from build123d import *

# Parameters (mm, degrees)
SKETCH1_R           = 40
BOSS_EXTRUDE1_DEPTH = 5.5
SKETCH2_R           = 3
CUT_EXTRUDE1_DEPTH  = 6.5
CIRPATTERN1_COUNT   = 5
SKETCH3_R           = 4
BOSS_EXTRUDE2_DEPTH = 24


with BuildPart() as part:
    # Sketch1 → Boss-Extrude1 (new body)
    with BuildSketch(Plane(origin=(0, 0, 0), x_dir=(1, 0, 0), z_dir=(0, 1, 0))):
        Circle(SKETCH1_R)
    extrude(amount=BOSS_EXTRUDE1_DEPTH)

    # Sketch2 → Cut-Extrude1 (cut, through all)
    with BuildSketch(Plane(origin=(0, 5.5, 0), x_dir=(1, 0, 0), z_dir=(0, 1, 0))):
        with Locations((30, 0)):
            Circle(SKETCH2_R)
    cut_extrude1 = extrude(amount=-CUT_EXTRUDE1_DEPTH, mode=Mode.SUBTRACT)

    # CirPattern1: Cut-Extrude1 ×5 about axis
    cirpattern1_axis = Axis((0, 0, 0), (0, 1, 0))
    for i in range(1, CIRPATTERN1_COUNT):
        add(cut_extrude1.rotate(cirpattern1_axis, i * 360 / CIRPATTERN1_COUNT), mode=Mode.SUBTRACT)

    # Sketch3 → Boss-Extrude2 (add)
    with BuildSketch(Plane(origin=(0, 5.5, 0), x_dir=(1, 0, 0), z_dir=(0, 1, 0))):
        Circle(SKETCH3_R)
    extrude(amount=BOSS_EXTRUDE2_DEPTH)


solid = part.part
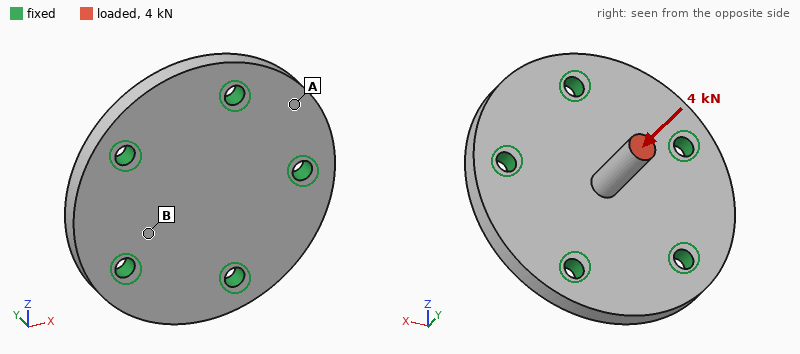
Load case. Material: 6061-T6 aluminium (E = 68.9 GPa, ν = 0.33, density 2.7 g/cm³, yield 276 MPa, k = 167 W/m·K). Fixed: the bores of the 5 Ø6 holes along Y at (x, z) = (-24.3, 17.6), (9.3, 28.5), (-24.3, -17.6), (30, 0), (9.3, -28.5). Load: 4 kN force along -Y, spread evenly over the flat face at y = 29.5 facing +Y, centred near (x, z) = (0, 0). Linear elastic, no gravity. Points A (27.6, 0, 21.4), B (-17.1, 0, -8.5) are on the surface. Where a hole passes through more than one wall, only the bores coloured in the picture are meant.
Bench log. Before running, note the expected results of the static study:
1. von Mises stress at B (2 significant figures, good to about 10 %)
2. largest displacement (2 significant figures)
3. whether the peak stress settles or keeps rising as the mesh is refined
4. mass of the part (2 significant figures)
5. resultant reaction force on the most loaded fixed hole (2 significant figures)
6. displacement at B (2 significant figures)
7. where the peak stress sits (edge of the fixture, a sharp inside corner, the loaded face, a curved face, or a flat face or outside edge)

32 MPa
0.10 mm
keeps rising
76 g
800 N
0.022 mm
edge of the fixture
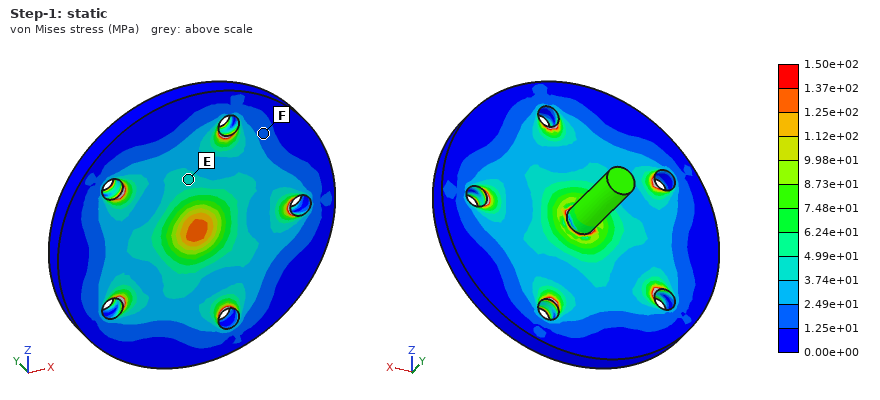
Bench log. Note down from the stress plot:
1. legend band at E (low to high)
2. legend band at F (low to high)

3.74e+01 to 4.99e+01 MPa
1.25e+01 to 2.49e+01 MPa
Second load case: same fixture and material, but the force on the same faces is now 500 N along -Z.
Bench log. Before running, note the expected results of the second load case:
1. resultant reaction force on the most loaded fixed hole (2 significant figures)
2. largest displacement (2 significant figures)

270 N
0.26 mm
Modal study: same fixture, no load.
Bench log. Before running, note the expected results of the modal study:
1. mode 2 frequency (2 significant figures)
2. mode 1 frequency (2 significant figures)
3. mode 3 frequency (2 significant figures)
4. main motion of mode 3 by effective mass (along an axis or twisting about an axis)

7300 Hz
7300 Hz
11 kHz
along Y
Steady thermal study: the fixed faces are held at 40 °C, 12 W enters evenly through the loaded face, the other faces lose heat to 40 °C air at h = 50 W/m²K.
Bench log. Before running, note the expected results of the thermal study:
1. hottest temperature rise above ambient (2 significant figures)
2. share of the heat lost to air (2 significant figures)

39 K
9.1 %
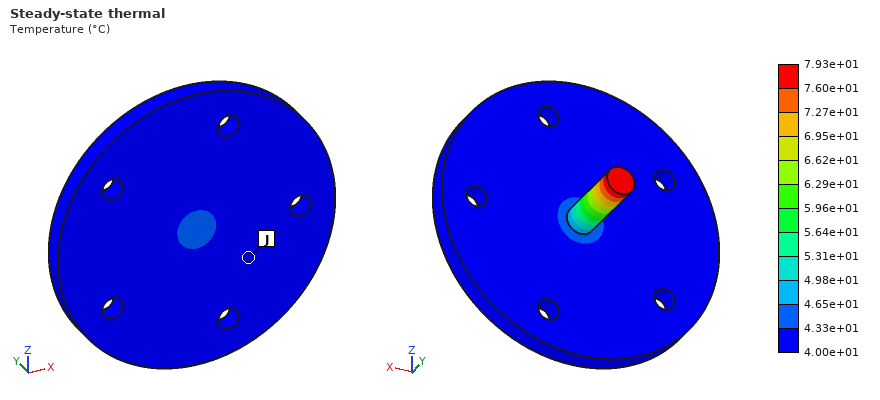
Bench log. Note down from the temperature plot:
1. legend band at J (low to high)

4.00e+01 to 4.33e+01 °C
